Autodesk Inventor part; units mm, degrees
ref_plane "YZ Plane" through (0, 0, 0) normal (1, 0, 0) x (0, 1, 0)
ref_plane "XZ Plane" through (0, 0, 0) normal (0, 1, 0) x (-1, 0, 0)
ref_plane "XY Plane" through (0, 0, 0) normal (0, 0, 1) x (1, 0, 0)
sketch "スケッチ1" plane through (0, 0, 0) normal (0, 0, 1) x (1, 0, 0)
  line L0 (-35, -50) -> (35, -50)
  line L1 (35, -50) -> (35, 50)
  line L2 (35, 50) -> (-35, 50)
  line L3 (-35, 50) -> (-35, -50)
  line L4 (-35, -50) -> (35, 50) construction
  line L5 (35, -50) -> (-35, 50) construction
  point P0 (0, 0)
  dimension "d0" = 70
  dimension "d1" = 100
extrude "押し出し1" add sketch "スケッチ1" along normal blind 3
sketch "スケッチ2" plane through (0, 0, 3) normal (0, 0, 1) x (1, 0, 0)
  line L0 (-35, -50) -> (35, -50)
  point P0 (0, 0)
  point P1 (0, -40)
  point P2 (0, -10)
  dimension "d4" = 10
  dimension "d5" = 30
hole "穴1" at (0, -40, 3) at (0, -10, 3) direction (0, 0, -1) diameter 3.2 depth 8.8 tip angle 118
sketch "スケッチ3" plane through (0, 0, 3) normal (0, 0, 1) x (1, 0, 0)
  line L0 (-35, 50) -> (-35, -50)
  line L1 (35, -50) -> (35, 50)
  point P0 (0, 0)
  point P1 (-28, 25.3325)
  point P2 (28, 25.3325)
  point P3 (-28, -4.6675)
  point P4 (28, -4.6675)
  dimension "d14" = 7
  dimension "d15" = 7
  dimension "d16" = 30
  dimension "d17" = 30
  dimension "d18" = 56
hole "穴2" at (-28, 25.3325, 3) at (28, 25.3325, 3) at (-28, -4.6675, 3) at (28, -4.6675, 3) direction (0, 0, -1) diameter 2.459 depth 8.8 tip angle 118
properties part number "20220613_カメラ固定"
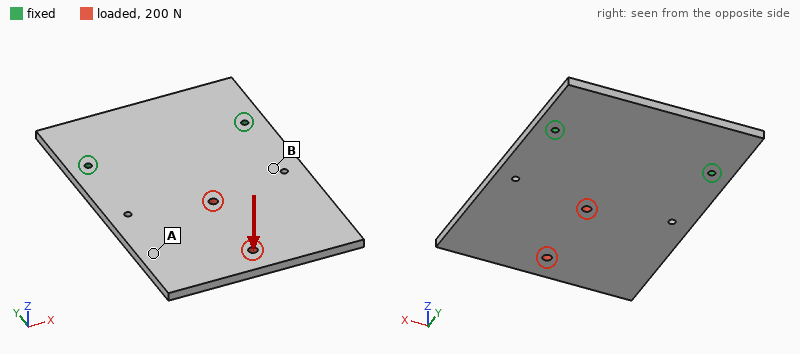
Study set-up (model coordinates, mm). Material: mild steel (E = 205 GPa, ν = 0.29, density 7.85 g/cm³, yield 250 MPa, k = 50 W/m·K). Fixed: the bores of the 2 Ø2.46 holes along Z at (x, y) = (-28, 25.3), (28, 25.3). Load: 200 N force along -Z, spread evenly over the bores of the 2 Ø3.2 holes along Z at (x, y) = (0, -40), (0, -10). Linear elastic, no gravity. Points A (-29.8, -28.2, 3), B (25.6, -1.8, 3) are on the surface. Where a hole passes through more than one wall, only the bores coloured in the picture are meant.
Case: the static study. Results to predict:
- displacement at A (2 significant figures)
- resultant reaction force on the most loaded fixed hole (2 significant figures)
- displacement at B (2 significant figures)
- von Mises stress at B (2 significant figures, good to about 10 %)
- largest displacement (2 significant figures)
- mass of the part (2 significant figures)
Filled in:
0.39 mm
100 N
0.14 mm
46 MPa
0.65 mm
160 g
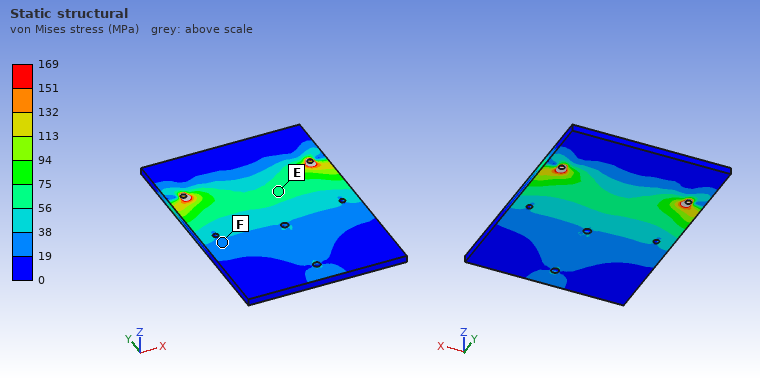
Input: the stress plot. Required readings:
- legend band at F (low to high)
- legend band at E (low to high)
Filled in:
19 to 38 MPa
56 to 75 MPa
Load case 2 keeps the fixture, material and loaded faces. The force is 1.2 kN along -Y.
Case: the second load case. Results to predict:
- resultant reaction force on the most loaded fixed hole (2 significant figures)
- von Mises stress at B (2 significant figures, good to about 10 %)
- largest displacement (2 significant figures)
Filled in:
600 N
6.2 MPa
3.1 µm
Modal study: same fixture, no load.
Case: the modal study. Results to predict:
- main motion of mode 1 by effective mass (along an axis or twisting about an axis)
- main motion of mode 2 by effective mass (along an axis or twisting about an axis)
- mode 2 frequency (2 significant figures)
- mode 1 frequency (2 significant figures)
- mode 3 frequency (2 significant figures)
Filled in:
along Z
twisting about Y
1100 Hz
380 Hz
2300 Hz
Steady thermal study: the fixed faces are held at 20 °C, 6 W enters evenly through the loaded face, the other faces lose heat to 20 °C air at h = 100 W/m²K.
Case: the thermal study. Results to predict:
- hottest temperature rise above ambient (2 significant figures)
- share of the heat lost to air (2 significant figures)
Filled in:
14 K
89 %
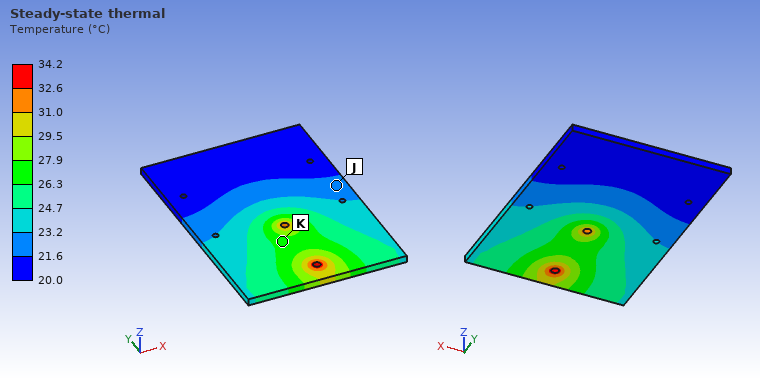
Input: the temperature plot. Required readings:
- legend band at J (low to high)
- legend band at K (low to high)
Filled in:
21.6 to 23.2 °C
26.3 to 27.9 °C
